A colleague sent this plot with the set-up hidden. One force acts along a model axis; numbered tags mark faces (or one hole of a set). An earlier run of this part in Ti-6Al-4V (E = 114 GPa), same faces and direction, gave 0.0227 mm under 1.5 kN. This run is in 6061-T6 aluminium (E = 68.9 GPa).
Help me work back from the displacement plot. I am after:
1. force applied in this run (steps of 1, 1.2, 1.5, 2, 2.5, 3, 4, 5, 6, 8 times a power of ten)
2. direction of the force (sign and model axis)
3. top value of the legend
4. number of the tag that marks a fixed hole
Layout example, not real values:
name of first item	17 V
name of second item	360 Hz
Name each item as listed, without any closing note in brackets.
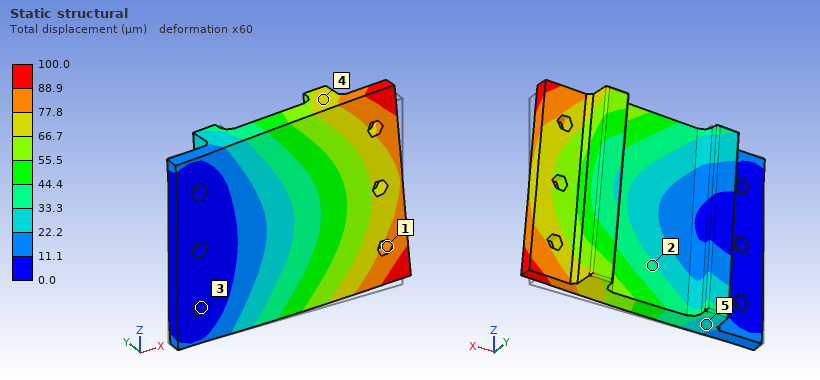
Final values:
force applied in this run	4 kN
direction of the force	+Z
top value of the legend	100.0 µm
number of the tag that marks a fixed hole	3
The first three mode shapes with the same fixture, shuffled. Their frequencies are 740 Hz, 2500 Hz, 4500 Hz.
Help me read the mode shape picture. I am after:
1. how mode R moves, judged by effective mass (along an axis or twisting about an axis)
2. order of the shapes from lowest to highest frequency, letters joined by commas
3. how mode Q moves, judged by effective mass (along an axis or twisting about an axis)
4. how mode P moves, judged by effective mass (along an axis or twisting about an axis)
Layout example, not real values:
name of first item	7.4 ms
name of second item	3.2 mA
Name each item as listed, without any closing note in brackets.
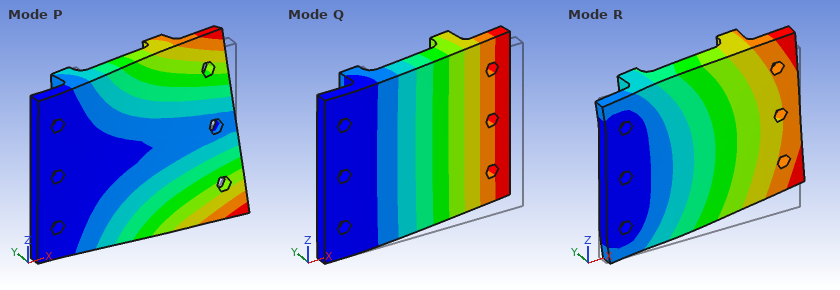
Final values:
how mode R moves, judged by effective mass	along Z
order of the shapes from lowest to highest frequency, letters joined by commas	Q, P, R
how mode Q moves, judged by effective mass	along Y
how mode P moves, judged by effective mass	twisting about X
